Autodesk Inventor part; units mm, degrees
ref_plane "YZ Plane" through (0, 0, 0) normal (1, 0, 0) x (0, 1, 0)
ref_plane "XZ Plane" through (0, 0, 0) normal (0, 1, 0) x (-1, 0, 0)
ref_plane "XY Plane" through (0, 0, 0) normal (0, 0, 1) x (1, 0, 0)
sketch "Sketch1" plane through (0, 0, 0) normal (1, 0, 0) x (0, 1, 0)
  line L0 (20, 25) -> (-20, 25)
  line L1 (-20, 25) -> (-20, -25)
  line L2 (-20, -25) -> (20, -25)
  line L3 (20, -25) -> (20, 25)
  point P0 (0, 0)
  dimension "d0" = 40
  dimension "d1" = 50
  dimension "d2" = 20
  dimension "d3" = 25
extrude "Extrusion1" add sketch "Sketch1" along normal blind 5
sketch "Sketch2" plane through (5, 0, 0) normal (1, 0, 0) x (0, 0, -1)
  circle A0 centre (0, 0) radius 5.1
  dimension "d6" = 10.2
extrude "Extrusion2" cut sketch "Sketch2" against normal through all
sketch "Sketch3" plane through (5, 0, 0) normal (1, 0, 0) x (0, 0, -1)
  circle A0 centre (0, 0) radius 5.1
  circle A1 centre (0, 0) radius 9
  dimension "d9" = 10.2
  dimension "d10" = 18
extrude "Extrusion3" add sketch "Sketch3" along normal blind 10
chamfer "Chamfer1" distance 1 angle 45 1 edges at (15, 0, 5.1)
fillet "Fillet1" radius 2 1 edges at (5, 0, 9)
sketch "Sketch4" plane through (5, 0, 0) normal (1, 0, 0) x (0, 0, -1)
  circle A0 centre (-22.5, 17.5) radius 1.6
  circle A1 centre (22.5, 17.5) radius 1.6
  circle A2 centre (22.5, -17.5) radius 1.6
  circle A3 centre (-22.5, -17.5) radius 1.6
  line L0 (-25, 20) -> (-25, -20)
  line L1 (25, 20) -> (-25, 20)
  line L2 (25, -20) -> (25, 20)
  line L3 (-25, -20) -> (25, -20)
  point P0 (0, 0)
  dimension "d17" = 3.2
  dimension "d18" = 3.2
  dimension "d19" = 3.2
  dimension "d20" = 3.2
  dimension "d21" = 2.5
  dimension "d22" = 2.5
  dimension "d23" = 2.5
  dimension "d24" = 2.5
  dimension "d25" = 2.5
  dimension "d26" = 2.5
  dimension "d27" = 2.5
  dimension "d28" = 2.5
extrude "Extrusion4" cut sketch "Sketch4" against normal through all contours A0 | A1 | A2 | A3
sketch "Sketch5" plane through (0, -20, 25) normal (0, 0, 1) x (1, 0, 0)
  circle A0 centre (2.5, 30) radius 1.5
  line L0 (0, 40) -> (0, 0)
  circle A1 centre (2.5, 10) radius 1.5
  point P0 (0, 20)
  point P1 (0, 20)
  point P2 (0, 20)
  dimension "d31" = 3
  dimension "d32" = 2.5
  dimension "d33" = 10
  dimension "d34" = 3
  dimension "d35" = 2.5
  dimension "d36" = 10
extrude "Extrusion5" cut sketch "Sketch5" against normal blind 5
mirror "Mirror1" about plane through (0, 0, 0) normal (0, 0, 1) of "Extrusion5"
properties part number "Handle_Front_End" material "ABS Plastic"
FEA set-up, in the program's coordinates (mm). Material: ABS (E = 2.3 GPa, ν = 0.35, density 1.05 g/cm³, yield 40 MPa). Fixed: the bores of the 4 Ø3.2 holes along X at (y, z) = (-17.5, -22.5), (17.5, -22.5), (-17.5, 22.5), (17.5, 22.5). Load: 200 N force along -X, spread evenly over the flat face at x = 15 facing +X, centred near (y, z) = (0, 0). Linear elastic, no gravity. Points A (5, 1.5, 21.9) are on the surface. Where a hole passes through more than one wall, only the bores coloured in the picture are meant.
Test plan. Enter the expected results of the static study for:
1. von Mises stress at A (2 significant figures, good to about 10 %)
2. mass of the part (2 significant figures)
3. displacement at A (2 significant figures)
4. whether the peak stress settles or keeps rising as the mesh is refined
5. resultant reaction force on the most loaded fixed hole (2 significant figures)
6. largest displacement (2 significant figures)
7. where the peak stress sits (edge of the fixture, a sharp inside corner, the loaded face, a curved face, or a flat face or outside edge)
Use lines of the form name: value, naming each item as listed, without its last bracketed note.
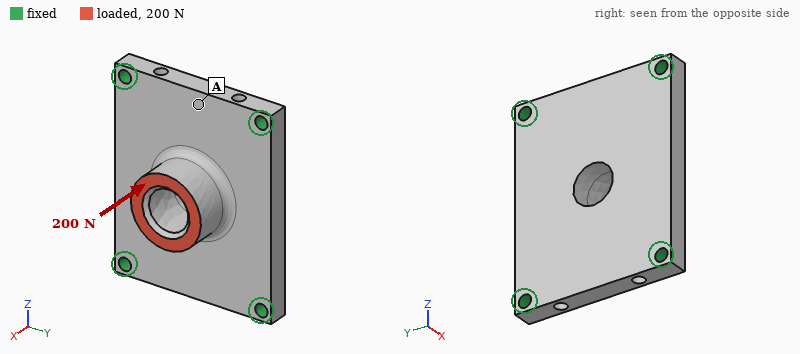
von Mises stress at A: 1.9 MPa
mass of the part: 12 g
displacement at A: 0.041 mm
whether the peak stress settles or keeps rising as the mesh is refined: keeps rising
resultant reaction force on the most loaded fixed hole: 52 N
largest displacement: 0.13 mm
where the peak stress sits: edge of the fixture
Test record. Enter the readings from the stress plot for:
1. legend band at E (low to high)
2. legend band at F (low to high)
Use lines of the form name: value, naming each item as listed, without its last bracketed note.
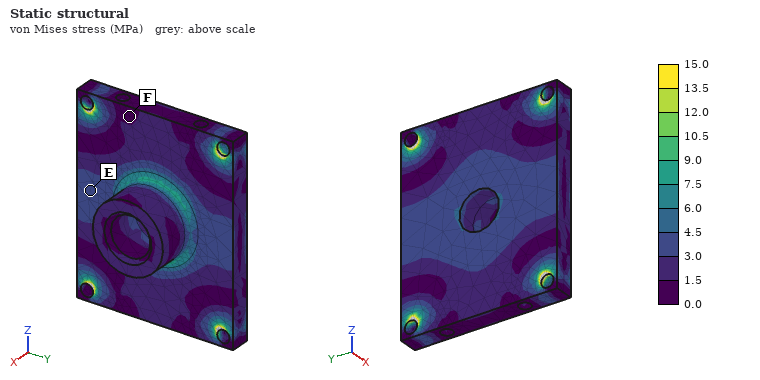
legend band at E: 3.0 to 4.5 MPa
legend band at F: 0.0 to 1.5 MPa
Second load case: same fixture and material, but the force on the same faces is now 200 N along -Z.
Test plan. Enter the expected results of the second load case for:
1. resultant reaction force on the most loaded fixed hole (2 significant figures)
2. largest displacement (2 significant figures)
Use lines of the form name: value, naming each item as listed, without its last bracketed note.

resultant reaction force on the most loaded fixed hole: 65 N
largest displacement: 0.13 mm
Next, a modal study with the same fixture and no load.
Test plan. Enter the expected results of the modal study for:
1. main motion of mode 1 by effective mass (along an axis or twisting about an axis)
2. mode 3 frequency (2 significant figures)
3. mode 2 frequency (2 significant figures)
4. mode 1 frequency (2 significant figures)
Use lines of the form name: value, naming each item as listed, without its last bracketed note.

main motion of mode 1 by effective mass: along X
mode 3 frequency: 4700 Hz
mode 2 frequency: 3800 Hz
mode 1 frequency: 2500 Hz
